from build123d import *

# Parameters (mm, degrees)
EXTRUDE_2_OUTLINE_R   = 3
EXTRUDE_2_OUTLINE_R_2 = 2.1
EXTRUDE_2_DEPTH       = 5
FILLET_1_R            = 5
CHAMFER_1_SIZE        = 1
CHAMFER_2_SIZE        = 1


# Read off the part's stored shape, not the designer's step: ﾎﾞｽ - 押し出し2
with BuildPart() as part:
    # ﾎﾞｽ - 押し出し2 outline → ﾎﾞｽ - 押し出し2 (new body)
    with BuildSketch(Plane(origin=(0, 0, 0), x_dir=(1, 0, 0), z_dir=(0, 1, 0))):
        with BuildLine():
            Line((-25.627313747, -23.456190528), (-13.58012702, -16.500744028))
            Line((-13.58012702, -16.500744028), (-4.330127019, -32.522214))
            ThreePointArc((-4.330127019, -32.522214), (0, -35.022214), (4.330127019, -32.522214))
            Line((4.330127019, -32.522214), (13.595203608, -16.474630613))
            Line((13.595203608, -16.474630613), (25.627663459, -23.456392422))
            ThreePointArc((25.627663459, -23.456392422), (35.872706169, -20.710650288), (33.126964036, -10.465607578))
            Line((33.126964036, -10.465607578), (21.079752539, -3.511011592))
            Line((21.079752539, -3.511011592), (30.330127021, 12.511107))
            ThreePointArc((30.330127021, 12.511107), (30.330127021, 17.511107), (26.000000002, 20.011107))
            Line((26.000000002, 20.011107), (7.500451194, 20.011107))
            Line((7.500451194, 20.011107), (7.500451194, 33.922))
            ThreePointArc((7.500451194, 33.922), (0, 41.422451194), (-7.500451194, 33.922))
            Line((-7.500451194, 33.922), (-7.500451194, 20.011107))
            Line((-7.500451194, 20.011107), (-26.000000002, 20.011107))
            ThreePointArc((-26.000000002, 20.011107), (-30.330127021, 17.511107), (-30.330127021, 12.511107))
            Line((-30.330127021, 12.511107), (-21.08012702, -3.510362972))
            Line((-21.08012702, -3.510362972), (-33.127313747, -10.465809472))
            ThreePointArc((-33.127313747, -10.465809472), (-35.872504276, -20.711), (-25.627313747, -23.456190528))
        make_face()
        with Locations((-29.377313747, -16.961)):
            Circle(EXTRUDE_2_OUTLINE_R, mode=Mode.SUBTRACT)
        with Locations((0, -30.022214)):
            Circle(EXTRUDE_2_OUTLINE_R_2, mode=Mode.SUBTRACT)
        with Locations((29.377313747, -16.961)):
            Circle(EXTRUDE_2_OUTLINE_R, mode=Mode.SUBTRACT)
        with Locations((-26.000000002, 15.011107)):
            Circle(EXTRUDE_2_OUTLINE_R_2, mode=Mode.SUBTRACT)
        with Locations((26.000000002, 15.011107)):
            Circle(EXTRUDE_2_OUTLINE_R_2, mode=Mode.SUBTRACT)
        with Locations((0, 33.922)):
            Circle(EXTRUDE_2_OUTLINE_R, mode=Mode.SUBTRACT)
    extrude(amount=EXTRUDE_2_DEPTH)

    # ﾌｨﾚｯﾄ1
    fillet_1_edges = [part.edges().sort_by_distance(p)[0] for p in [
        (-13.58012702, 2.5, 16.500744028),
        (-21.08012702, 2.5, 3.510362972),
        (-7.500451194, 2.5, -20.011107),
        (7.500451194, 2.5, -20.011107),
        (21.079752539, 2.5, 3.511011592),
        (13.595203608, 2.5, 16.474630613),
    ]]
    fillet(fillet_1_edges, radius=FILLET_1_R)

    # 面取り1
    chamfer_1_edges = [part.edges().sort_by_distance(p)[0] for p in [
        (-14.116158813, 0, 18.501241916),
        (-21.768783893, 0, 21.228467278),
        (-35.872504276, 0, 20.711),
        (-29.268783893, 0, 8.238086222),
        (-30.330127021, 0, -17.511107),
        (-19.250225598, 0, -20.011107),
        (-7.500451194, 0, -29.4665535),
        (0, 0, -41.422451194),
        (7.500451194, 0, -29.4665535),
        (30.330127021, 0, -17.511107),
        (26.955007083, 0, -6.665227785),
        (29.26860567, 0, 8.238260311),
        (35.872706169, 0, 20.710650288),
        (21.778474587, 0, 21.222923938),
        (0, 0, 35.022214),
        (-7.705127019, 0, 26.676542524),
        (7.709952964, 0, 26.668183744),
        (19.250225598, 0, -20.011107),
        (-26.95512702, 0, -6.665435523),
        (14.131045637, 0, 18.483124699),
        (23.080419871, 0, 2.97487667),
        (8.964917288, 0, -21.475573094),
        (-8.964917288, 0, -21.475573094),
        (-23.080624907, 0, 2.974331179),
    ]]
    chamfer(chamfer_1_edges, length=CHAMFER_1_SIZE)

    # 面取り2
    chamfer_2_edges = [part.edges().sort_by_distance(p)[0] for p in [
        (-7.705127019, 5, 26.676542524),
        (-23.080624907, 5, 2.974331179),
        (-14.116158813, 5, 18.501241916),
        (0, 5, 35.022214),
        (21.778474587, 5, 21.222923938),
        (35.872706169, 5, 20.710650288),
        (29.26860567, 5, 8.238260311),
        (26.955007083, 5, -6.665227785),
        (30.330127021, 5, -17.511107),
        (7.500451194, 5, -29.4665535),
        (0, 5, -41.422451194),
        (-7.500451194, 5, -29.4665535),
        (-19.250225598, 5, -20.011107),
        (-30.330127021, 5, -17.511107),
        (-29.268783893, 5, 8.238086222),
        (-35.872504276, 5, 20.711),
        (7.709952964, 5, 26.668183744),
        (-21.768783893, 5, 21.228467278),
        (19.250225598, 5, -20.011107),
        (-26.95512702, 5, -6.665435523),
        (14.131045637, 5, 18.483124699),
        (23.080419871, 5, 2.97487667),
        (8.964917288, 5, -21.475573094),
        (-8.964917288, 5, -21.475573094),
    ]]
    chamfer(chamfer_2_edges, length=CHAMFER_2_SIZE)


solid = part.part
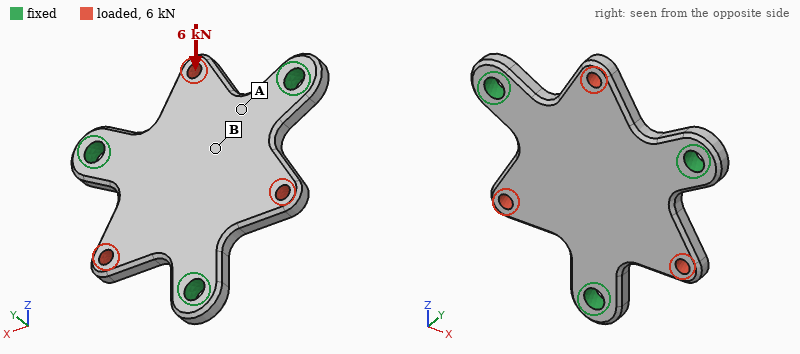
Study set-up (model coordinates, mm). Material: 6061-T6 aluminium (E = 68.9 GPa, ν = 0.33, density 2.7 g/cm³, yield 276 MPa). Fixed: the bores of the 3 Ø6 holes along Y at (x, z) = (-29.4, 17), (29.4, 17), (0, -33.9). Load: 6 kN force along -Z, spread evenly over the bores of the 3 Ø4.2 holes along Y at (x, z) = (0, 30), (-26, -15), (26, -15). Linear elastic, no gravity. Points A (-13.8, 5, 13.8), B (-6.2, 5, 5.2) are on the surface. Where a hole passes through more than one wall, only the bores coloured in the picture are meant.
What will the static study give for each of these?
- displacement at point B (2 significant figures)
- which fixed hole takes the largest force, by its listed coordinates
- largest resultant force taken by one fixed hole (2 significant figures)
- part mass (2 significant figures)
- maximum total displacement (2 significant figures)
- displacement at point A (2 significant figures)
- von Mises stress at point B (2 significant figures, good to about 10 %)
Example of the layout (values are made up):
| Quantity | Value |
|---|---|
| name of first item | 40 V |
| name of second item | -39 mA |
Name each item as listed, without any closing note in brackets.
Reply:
| Quantity | Value |
|---|---|
| displacement at point B | 15 µm |
| which fixed hole takes the largest force, by its listed coordinates | (0, -33.9) |
| largest resultant force taken by one fixed hole | 2.7 kN |
| part mass | 37 g |
| maximum total displacement | 41 µm |
| displacement at point A | 15 µm |
| von Mises stress at point B | 32 MPa |
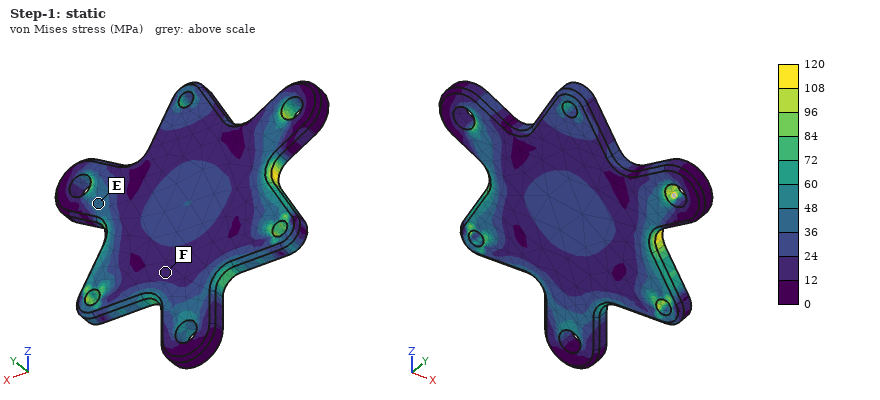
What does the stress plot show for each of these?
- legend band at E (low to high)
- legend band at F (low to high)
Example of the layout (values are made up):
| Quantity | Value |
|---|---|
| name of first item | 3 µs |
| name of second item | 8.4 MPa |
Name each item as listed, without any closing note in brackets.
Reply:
| Quantity | Value |
|---|---|
| legend band at E | 36 to 48 MPa |
| legend band at F | 12 to 24 MPa |
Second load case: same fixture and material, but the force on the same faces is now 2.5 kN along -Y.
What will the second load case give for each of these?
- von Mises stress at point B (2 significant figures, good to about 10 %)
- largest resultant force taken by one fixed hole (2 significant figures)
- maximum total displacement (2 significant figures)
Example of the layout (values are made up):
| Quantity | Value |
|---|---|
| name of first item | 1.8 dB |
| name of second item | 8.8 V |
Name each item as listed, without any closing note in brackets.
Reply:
| Quantity | Value |
|---|---|
| von Mises stress at point B | 57 MPa |
| largest resultant force taken by one fixed hole | 830 N |
| maximum total displacement | 0.27 mm |
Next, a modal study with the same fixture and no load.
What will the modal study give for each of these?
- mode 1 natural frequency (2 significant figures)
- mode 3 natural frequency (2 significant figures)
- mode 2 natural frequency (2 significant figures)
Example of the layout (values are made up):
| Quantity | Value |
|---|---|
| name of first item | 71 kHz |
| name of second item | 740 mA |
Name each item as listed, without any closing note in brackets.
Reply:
| Quantity | Value |
|---|---|
| mode 1 natural frequency | 5800 Hz |
| mode 3 natural frequency | 6000 Hz |
| mode 2 natural frequency | 6000 Hz |
